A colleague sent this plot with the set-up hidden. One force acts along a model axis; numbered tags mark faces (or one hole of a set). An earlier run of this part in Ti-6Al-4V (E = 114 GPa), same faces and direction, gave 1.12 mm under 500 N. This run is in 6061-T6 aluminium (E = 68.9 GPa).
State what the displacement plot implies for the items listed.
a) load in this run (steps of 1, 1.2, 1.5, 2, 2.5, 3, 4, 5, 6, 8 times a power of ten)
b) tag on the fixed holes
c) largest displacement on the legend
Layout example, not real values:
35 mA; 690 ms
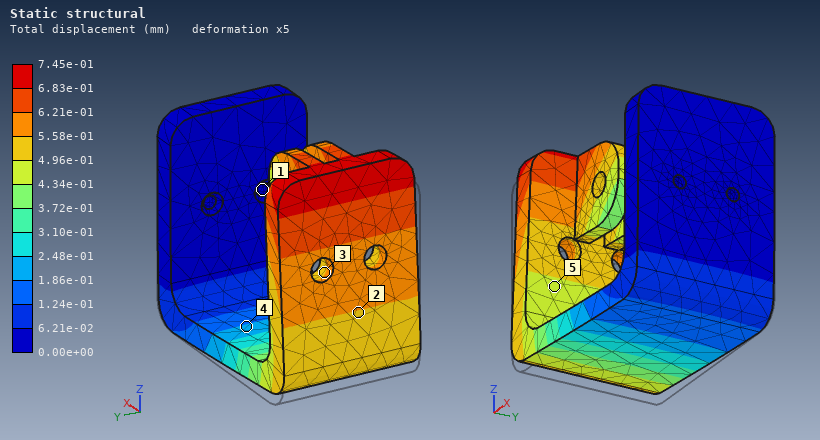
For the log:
200 N; 1; 7.45e-01 mm
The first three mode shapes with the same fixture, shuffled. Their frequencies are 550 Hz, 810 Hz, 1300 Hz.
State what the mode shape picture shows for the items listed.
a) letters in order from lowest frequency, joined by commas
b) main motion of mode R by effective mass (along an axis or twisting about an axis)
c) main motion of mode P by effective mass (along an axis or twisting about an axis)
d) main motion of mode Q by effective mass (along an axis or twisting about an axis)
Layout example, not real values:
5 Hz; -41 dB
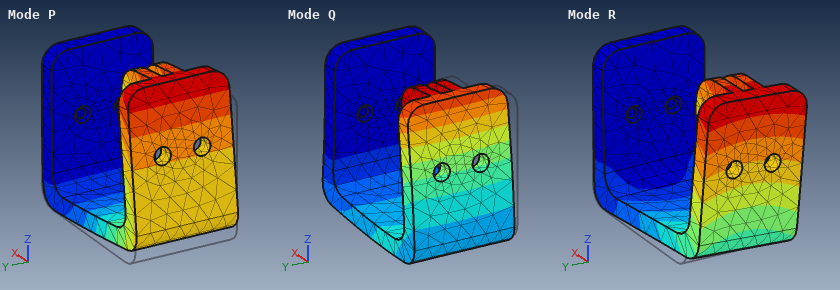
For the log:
P, R, Q; along Y; along Z; along X
